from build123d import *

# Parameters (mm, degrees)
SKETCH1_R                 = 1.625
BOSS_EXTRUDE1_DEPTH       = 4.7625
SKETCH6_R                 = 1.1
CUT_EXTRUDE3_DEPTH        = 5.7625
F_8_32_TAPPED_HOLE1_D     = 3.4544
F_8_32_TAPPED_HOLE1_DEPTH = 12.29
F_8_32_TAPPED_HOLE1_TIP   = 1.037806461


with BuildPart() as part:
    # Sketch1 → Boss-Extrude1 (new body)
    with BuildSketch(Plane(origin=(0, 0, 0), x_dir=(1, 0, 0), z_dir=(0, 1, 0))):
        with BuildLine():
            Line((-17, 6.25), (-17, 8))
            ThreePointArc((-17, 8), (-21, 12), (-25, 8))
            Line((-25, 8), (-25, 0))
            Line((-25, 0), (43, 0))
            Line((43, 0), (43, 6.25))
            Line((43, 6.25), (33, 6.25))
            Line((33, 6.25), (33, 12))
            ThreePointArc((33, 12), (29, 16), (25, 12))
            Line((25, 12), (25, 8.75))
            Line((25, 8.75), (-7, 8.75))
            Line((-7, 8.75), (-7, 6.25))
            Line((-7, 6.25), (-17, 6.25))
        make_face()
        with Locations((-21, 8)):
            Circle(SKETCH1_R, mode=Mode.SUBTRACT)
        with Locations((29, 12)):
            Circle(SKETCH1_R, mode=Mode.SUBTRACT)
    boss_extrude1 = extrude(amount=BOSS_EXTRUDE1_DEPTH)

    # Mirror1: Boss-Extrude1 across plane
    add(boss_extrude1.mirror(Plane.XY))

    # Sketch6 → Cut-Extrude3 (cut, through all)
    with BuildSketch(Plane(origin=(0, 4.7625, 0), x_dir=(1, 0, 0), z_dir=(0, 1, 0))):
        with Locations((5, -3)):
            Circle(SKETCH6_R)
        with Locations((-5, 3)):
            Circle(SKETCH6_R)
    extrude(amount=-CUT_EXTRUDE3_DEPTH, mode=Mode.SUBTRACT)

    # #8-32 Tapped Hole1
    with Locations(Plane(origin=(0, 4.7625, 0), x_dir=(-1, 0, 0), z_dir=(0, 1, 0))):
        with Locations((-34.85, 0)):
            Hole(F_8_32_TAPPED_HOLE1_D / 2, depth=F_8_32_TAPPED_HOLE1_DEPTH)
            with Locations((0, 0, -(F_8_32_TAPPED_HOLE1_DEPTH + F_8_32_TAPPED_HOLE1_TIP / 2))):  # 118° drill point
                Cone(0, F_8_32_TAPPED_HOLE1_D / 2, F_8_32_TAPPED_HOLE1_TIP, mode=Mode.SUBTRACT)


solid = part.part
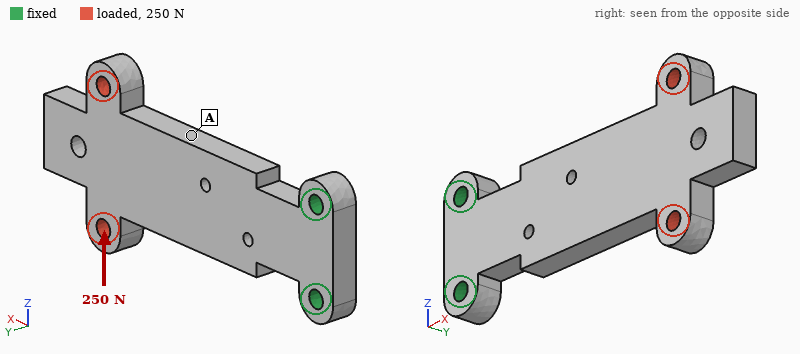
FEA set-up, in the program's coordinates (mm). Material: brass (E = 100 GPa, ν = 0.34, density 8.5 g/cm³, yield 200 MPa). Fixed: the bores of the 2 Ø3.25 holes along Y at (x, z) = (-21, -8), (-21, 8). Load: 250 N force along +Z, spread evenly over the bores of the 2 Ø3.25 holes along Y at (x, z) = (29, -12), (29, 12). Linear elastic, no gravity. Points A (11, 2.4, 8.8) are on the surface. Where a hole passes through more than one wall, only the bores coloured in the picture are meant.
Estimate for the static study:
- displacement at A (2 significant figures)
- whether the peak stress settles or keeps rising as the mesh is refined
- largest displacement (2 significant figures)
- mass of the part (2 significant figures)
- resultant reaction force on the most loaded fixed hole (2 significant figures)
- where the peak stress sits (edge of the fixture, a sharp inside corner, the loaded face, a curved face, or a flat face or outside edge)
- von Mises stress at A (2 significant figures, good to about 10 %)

0.061 mm
keeps rising
0.15 mm
48 g
870 N
a sharp inside corner
19 MPa
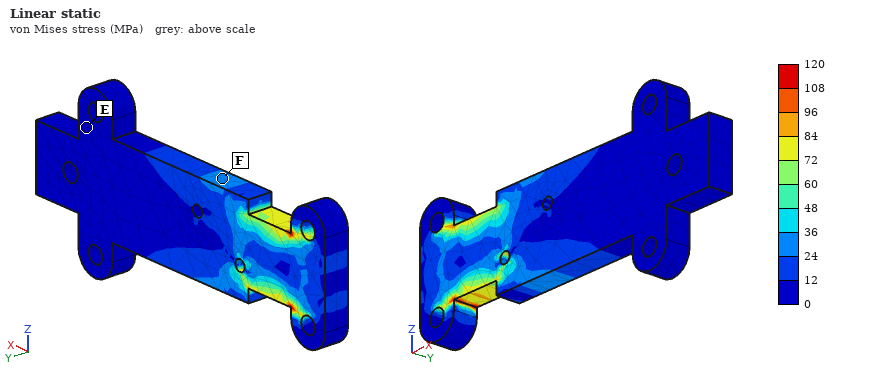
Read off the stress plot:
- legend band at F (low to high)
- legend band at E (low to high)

24 to 36 MPa
0 to 12 MPa
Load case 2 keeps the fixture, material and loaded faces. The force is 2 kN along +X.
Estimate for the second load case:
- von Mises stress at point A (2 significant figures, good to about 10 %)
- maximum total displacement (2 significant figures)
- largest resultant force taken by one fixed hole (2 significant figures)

25 MPa
31 µm
1.1 kN
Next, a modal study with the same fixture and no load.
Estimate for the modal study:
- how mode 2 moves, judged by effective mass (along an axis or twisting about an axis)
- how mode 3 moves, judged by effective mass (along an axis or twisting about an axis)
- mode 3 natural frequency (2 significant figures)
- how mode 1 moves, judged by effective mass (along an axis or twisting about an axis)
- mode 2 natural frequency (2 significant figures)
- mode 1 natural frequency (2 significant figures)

along Z
twisting about X
3000 Hz
along Y
1600 Hz
560 Hz
